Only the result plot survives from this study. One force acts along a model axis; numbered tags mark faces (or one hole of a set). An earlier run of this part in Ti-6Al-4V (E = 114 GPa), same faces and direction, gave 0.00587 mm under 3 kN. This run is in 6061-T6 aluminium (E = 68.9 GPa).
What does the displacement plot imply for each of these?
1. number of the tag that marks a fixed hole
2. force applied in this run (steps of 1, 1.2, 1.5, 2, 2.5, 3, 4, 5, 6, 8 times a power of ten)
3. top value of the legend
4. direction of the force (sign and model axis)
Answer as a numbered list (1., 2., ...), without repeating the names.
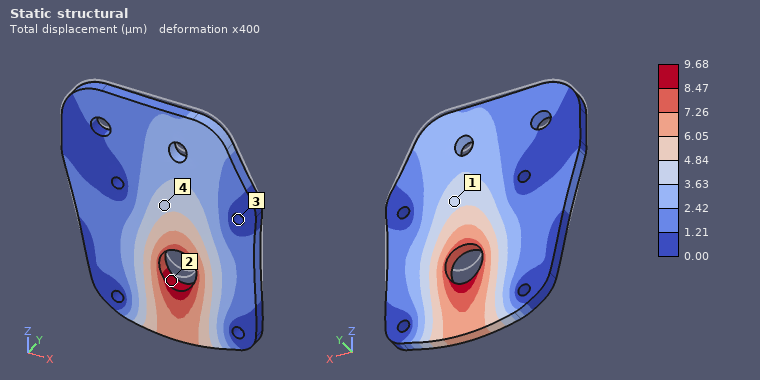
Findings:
1. 3
2. 3 kN
3. 9.68 µm
4. -Z
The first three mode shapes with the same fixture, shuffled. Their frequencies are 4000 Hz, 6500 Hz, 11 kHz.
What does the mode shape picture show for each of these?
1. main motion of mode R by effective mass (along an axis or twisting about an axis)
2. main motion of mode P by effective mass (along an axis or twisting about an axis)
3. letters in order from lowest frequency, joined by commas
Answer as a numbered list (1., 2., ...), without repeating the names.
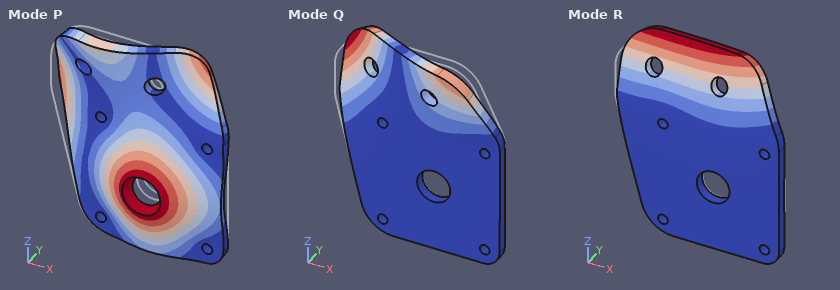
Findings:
1. along Y
2. along Y
3. R, Q, P
